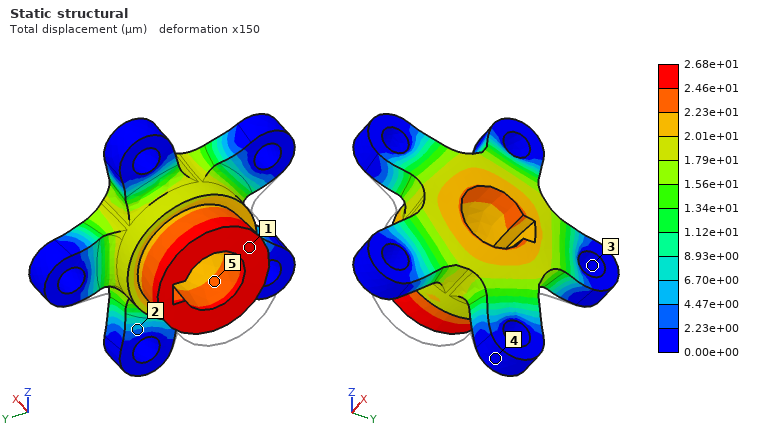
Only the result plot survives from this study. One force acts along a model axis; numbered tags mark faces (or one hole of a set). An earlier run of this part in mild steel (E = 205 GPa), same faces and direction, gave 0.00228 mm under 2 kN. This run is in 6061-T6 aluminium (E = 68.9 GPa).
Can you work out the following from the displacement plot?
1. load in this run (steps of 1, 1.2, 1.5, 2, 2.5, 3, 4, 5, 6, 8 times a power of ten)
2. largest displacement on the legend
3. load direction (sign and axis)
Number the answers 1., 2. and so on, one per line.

1. 8 kN
2. 2.68e+01 µm
3. +X
